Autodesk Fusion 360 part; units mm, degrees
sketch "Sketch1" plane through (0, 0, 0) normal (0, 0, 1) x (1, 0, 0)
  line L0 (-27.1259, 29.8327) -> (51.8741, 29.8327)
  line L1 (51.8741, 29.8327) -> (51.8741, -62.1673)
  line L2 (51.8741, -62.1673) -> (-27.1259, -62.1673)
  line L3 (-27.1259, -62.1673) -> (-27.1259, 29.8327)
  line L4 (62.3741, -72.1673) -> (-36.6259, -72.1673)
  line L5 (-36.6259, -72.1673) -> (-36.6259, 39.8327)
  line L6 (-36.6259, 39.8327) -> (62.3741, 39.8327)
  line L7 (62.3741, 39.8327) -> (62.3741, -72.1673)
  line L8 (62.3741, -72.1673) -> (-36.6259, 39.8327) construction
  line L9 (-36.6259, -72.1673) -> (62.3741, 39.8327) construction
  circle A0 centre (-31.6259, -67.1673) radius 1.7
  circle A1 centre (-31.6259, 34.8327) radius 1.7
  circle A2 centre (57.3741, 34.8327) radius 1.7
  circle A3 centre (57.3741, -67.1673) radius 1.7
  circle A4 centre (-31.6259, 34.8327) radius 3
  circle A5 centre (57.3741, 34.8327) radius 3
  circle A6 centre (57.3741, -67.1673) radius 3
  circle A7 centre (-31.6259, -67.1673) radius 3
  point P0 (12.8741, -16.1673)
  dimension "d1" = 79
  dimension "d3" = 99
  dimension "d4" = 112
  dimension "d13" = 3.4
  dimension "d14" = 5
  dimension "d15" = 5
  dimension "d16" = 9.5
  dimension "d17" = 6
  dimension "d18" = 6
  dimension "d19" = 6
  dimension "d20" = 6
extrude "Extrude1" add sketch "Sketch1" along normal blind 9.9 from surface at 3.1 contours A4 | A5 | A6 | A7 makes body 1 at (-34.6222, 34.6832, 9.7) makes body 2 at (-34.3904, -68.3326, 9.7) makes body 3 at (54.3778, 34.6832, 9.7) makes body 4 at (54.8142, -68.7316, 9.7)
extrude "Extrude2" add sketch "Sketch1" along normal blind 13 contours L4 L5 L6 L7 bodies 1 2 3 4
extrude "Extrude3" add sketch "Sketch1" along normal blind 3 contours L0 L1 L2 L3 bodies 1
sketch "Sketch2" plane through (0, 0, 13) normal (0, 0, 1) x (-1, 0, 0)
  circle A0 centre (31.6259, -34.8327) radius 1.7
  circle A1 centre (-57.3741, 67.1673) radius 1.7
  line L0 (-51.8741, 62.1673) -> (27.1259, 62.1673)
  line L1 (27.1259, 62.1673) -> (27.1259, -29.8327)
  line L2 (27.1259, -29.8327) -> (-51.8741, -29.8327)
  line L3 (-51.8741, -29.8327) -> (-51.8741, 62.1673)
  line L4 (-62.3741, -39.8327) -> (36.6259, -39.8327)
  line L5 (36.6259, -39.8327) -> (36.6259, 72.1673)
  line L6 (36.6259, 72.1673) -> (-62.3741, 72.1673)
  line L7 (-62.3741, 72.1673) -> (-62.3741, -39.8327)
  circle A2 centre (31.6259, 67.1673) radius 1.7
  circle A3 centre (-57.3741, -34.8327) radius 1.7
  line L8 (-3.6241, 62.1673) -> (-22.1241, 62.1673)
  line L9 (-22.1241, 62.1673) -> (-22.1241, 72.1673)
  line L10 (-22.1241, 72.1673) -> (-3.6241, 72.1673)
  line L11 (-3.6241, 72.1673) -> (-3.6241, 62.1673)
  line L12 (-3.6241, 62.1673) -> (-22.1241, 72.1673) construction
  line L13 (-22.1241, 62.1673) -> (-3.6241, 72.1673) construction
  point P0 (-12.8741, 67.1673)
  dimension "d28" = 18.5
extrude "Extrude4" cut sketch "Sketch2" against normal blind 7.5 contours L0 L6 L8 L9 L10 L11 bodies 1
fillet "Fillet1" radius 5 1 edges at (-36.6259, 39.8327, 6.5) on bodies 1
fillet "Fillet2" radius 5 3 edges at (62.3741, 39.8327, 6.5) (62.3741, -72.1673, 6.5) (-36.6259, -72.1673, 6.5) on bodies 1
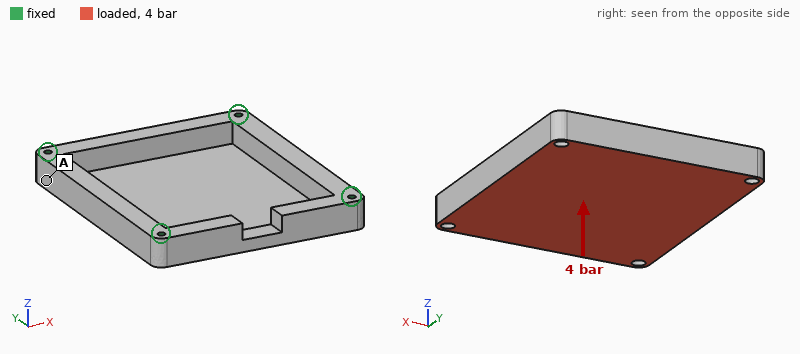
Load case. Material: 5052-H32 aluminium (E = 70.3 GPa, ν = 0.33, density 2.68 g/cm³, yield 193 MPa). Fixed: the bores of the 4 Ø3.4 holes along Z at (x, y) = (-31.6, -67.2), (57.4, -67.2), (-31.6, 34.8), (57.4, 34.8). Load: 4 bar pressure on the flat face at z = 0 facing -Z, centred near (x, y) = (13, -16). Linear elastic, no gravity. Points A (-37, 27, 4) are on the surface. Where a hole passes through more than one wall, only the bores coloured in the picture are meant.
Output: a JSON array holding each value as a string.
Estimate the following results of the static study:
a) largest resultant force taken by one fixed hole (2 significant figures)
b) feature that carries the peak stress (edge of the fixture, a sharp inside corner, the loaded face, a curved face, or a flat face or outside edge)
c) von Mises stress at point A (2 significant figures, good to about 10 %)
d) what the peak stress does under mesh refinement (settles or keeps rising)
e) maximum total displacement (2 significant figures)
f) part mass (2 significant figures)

["1.9 kN", "edge of the fixture", "12 MPa", "keeps rising", "0.26 mm", "190 g"]
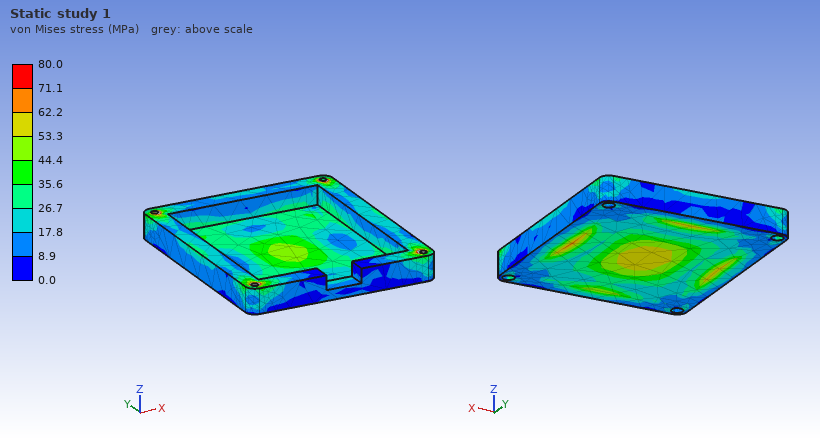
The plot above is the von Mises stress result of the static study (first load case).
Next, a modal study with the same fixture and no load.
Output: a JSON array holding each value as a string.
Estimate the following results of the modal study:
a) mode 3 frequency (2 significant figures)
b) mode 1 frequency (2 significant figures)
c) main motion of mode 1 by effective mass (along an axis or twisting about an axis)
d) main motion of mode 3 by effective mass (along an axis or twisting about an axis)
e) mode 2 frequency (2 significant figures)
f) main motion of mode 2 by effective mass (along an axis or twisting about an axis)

["5000 Hz", "2800 Hz", "along Z", "twisting about X", "4700 Hz", "twisting about Y"]
